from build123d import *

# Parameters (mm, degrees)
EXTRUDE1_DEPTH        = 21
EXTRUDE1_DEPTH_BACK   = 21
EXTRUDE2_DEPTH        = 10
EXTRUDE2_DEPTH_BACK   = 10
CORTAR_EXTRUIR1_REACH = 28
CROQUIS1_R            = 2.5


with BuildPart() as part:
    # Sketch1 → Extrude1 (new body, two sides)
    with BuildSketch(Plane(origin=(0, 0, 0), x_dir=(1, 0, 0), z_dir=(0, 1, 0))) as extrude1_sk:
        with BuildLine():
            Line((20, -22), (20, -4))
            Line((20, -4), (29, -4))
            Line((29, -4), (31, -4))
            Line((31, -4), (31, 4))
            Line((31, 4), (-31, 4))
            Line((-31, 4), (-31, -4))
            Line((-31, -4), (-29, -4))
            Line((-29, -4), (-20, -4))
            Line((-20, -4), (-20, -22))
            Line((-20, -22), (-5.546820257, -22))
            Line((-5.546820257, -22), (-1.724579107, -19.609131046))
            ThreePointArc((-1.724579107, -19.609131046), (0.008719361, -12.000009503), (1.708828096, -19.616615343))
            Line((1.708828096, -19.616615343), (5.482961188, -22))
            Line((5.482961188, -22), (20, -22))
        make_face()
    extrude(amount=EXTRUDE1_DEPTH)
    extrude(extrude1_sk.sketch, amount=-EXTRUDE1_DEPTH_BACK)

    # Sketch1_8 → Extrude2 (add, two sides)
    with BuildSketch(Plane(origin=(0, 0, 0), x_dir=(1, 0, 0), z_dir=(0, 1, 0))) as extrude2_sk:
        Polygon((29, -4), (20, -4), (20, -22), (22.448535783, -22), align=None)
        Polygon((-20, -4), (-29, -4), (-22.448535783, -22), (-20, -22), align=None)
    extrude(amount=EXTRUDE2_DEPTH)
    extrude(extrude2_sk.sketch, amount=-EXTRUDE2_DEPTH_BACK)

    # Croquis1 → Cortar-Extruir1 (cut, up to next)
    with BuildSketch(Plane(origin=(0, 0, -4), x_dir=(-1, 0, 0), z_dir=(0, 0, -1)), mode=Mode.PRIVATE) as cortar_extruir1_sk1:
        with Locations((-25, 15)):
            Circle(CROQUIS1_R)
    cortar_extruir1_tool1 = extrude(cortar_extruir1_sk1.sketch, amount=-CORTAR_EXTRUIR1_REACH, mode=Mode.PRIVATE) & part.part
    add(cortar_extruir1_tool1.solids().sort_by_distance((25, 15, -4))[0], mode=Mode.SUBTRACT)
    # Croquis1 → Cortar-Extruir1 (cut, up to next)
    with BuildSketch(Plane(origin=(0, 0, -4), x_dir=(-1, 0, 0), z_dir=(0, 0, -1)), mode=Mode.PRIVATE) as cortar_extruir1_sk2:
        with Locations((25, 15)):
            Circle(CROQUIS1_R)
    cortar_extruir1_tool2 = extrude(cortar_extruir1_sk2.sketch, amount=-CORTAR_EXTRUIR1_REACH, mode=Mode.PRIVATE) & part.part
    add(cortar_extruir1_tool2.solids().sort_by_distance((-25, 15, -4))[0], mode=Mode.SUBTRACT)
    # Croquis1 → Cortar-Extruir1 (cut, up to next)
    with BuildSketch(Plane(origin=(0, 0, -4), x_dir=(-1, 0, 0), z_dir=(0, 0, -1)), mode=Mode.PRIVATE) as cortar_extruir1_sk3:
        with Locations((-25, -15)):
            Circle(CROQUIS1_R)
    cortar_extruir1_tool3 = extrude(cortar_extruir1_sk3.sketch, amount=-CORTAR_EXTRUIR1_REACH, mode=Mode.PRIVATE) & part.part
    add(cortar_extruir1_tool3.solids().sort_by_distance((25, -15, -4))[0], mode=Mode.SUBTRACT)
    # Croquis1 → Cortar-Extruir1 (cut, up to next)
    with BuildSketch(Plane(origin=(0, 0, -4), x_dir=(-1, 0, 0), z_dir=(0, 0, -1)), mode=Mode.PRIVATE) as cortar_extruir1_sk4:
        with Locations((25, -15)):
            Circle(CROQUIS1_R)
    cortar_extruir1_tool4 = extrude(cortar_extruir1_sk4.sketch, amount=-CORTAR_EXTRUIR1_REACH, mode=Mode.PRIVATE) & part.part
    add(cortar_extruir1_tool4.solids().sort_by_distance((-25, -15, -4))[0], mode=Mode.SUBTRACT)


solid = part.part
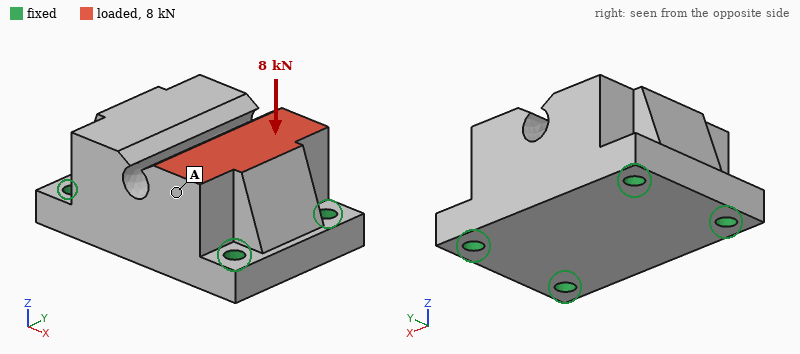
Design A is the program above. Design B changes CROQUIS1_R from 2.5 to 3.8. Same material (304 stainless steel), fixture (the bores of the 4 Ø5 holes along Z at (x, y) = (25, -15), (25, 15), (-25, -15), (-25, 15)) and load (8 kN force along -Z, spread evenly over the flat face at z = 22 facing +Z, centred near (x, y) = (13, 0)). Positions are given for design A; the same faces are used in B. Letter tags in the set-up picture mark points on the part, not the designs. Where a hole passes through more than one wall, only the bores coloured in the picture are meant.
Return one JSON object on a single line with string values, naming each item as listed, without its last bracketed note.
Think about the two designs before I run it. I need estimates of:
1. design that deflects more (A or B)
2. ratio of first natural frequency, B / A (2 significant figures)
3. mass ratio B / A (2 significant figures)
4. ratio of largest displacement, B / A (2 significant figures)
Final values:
{"design that deflects more": "A", "ratio of first natural frequency, B / A": "1.1", "mass ratio B / A": "0.98", "ratio of largest displacement, B / A": "0.81"}
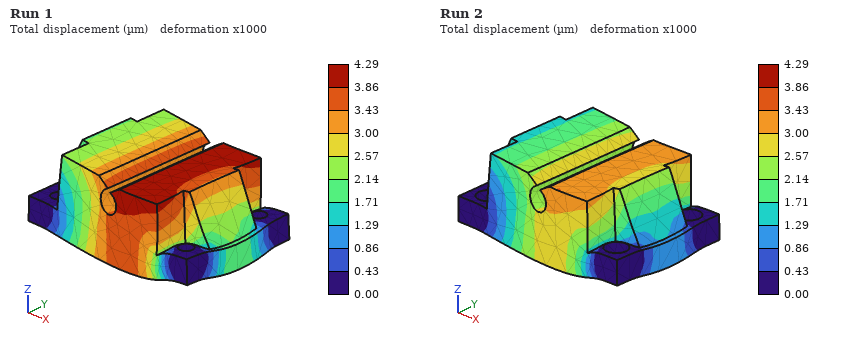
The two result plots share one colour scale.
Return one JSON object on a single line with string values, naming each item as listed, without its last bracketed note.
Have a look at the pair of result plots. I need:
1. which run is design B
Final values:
{"which run is design B": "Run 2"}
